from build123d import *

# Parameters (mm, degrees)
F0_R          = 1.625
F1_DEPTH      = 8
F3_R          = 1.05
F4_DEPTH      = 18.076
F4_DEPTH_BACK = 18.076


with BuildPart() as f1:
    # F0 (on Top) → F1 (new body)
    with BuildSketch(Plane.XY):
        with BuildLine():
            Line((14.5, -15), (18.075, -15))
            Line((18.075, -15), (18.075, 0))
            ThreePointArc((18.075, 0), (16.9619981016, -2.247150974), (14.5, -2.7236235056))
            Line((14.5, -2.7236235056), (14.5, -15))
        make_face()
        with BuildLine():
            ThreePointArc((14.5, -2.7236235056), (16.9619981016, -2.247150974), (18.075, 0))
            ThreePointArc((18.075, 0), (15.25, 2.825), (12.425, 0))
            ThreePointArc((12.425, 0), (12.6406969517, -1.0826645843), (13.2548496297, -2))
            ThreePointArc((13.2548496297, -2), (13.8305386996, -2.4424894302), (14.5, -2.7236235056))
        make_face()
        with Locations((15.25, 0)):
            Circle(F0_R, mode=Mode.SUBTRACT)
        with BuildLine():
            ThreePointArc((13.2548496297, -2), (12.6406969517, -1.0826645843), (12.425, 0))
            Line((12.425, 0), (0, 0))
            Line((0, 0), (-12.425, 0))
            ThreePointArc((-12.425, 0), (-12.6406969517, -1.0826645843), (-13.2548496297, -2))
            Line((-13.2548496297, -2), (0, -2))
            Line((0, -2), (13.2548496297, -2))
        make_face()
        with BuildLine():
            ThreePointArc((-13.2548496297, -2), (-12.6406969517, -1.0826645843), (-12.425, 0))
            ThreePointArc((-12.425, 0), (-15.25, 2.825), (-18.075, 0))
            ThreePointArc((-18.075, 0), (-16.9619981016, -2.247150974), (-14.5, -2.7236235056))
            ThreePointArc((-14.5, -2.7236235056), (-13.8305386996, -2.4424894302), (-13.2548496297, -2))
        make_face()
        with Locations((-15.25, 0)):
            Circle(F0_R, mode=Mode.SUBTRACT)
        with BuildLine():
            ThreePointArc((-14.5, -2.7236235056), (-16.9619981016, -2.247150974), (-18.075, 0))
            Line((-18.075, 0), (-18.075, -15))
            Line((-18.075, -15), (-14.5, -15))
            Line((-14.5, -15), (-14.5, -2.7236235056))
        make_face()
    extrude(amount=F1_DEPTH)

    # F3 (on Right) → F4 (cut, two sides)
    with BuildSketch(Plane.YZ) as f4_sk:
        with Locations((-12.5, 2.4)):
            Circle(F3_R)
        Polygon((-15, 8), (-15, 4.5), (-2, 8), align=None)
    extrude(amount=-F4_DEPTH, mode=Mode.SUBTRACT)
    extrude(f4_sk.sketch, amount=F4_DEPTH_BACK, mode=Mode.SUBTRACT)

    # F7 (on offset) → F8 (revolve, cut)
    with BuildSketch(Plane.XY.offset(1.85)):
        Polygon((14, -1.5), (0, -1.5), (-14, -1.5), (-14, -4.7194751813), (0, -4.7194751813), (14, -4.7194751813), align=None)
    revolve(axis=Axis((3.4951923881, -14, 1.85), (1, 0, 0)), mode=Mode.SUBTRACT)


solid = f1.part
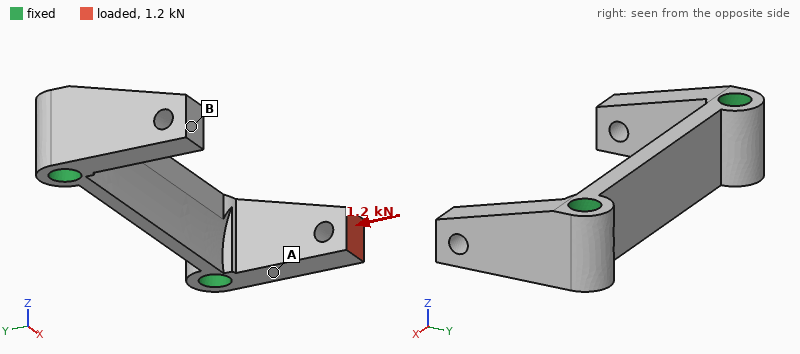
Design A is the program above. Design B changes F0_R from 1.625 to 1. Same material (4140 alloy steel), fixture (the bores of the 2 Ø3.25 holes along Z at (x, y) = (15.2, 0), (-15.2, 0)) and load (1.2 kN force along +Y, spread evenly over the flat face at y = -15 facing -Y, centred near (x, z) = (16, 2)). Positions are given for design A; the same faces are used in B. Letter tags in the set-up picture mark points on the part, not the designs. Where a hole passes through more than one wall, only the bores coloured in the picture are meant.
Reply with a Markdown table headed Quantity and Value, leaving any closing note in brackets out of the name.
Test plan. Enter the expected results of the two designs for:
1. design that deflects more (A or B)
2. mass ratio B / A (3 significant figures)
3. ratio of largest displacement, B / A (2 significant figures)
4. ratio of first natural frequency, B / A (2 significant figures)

| Quantity | Value |
|---|---|
| design that deflects more | B |
| mass ratio B / A | 1.07 |
| ratio of largest displacement, B / A | 1.1 |
| ratio of first natural frequency, B / A | 0.97 |
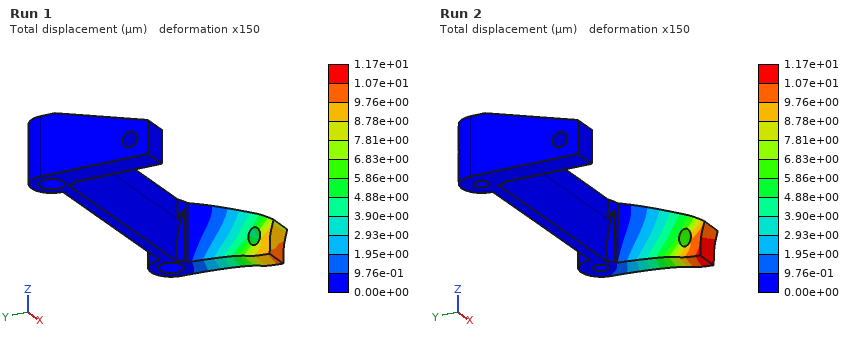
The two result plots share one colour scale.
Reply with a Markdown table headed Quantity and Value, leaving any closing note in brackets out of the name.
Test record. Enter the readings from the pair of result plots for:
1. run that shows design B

| Quantity | Value |
|---|---|
| run that shows design B | Run 2 |
